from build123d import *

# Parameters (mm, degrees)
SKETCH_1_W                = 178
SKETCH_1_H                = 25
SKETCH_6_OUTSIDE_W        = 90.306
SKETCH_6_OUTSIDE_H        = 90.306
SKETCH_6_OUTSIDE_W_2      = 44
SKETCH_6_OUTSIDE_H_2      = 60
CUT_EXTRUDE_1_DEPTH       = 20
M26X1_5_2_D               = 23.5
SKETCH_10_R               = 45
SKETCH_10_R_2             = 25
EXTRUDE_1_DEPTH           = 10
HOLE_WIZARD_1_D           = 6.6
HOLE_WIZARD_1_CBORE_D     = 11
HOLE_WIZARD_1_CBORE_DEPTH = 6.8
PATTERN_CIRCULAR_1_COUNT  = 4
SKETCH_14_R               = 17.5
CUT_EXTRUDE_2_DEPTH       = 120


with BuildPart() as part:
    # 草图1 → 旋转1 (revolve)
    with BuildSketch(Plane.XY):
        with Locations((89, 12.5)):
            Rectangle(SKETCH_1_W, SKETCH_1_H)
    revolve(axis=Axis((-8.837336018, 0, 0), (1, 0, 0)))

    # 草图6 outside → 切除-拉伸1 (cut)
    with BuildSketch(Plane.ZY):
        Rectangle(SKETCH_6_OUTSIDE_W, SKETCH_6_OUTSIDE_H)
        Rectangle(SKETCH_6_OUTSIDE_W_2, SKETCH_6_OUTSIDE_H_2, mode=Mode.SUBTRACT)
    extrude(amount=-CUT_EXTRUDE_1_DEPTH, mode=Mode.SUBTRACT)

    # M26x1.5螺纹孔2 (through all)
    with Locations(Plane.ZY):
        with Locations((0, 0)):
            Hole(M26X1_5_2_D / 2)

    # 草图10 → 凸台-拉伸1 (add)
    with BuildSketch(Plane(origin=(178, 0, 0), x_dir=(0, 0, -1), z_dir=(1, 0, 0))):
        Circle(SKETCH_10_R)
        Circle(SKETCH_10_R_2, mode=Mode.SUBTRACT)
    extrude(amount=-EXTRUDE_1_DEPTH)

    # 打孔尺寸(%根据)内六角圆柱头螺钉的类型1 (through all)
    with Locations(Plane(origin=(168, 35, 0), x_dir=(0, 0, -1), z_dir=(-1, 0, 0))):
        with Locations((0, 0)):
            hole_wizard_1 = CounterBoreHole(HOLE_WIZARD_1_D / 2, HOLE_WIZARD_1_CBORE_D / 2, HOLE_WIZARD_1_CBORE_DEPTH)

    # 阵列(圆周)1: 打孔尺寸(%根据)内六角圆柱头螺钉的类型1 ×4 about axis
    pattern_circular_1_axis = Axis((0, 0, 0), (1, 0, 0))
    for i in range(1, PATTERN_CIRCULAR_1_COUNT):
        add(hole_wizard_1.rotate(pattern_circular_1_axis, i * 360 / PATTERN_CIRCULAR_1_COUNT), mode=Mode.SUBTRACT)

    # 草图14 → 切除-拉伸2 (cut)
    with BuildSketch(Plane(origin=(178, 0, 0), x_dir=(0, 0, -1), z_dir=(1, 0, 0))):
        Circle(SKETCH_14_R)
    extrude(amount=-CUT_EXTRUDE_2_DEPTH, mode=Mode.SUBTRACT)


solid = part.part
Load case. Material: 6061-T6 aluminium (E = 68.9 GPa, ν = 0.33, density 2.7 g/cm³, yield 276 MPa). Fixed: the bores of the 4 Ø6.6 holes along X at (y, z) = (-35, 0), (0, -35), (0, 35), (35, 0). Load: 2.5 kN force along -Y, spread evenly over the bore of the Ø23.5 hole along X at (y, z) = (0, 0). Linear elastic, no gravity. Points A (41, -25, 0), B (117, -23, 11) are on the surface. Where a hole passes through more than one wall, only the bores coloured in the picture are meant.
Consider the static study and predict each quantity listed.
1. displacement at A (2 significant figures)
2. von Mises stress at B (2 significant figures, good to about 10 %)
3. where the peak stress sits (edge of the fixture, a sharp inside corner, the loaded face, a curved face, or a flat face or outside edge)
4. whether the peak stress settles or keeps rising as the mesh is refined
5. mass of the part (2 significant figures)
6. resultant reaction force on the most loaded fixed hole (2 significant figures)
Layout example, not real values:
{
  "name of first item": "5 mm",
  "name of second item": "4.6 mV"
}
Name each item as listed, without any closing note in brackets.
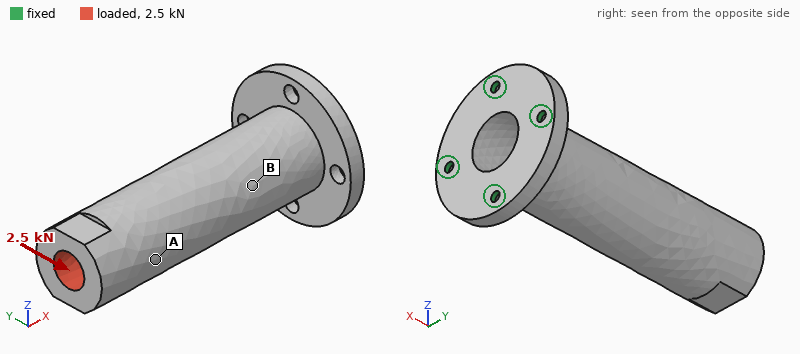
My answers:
{
  "displacement at A": "0.32 mm",
  "von Mises stress at B": "21 MPa",
  "where the peak stress sits": "edge of the fixture",
  "whether the peak stress settles or keeps rising as the mesh is refined": "keeps rising",
  "mass of the part": "670 g",
  "resultant reaction force on the most loaded fixed hole": "6.1 kN"
}
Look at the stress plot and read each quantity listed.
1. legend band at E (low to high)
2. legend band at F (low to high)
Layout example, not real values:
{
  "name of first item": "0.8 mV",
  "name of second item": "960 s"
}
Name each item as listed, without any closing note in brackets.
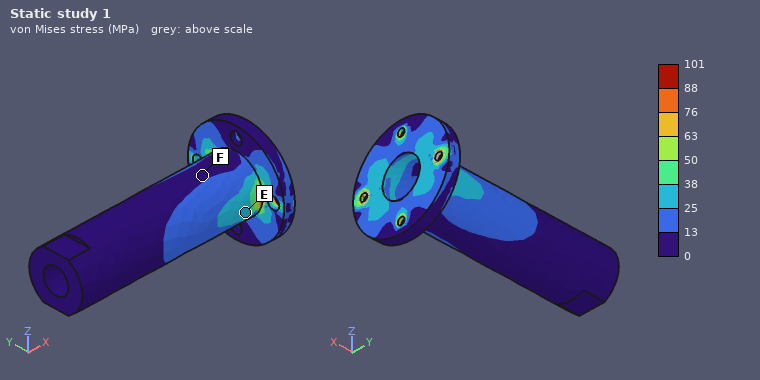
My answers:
{
  "legend band at E": "25 to 38 MPa",
  "legend band at F": "0 to 13 MPa"
}
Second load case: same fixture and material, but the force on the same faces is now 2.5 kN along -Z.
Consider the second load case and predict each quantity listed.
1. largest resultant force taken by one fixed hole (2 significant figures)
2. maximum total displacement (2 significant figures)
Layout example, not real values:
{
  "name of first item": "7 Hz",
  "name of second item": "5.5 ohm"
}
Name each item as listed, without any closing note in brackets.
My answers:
{
  "largest resultant force taken by one fixed hole": "6.1 kN",
  "maximum total displacement": "0.43 mm"
}
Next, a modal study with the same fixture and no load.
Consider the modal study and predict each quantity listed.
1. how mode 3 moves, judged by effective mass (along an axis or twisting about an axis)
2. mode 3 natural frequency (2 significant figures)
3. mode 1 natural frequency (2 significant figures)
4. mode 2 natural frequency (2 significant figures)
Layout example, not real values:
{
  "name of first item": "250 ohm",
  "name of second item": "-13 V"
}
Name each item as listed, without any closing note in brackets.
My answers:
{
  "how mode 3 moves, judged by effective mass": "along X",
  "mode 3 natural frequency": "4100 Hz",
  "mode 1 natural frequency": "790 Hz",
  "mode 2 natural frequency": "790 Hz"
}
